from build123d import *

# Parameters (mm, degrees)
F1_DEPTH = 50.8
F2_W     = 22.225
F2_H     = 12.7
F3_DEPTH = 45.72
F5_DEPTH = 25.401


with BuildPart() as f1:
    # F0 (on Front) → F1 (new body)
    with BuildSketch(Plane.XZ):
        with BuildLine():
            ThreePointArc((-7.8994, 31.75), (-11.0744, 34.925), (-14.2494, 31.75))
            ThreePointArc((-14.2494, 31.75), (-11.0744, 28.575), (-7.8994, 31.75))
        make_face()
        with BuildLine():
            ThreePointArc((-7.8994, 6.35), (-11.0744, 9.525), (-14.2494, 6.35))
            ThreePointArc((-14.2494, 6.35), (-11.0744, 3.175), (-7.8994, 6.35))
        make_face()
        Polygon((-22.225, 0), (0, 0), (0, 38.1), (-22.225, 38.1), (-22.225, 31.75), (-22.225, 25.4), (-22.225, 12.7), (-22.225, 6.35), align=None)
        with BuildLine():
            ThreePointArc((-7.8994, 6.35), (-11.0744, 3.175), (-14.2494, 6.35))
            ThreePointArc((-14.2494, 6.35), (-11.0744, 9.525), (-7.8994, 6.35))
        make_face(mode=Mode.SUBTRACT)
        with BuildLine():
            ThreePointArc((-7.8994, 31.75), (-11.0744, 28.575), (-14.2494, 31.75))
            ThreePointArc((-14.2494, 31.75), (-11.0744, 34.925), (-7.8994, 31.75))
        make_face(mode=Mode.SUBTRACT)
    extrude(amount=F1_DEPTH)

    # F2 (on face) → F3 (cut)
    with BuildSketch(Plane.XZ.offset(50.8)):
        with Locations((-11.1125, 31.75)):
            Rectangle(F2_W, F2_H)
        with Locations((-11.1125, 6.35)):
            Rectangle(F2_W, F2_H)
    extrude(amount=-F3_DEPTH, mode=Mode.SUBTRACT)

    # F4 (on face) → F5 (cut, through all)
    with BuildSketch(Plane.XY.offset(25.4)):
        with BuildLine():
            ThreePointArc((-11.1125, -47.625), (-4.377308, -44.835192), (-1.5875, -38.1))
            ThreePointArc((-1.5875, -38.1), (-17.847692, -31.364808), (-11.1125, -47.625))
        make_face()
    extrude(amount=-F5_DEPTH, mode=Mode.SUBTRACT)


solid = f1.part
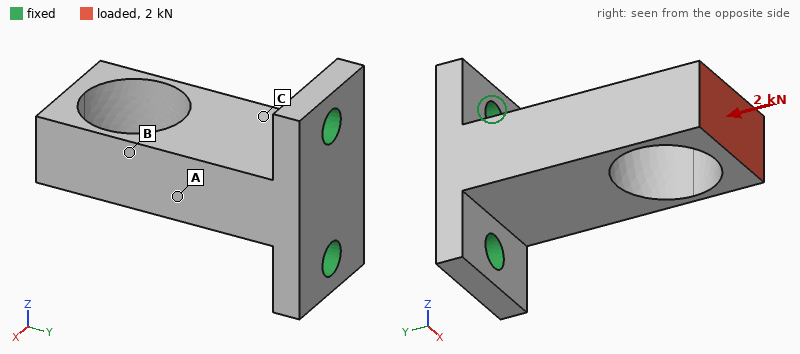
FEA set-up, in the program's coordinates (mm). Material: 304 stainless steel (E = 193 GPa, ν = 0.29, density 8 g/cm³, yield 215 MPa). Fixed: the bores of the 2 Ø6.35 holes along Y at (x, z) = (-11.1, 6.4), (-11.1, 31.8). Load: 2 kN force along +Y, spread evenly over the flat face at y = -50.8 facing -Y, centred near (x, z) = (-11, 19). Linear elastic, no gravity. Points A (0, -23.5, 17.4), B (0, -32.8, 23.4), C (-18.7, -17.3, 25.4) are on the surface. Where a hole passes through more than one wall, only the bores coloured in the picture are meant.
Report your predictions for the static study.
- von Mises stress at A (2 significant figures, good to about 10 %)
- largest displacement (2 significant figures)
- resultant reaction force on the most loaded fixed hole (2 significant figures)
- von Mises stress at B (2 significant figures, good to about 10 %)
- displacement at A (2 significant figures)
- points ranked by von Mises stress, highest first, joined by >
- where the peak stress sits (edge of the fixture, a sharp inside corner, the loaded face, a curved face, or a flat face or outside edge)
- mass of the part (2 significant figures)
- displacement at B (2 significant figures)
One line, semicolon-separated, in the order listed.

29 MPa; 20 µm; 1.0 kN; 81 MPa; 3.1 µm; B > A > C; a curved face; 110 g; 6.4 µm
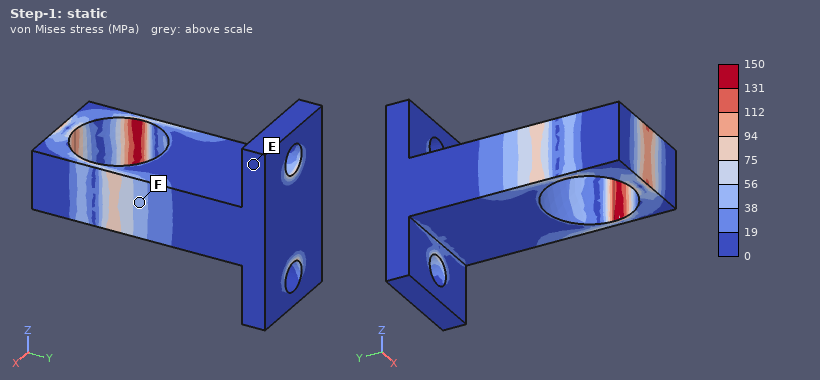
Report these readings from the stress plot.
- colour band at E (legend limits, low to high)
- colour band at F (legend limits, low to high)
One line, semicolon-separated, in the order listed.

0 to 19 MPa; 38 to 56 MPa
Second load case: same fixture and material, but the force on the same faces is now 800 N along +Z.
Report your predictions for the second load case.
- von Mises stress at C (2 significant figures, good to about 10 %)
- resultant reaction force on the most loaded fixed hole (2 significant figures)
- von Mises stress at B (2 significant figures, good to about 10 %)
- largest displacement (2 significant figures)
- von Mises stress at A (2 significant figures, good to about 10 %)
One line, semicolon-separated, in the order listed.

46 MPa; 2.1 kN; 84 MPa; 85 µm; 15 MPa
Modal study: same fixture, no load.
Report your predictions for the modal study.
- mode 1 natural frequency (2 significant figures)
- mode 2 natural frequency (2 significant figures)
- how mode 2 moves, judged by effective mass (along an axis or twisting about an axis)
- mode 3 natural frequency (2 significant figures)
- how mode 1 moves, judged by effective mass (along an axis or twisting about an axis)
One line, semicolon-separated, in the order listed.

3200 Hz; 4200 Hz; along Z; 10 kHz; along X
